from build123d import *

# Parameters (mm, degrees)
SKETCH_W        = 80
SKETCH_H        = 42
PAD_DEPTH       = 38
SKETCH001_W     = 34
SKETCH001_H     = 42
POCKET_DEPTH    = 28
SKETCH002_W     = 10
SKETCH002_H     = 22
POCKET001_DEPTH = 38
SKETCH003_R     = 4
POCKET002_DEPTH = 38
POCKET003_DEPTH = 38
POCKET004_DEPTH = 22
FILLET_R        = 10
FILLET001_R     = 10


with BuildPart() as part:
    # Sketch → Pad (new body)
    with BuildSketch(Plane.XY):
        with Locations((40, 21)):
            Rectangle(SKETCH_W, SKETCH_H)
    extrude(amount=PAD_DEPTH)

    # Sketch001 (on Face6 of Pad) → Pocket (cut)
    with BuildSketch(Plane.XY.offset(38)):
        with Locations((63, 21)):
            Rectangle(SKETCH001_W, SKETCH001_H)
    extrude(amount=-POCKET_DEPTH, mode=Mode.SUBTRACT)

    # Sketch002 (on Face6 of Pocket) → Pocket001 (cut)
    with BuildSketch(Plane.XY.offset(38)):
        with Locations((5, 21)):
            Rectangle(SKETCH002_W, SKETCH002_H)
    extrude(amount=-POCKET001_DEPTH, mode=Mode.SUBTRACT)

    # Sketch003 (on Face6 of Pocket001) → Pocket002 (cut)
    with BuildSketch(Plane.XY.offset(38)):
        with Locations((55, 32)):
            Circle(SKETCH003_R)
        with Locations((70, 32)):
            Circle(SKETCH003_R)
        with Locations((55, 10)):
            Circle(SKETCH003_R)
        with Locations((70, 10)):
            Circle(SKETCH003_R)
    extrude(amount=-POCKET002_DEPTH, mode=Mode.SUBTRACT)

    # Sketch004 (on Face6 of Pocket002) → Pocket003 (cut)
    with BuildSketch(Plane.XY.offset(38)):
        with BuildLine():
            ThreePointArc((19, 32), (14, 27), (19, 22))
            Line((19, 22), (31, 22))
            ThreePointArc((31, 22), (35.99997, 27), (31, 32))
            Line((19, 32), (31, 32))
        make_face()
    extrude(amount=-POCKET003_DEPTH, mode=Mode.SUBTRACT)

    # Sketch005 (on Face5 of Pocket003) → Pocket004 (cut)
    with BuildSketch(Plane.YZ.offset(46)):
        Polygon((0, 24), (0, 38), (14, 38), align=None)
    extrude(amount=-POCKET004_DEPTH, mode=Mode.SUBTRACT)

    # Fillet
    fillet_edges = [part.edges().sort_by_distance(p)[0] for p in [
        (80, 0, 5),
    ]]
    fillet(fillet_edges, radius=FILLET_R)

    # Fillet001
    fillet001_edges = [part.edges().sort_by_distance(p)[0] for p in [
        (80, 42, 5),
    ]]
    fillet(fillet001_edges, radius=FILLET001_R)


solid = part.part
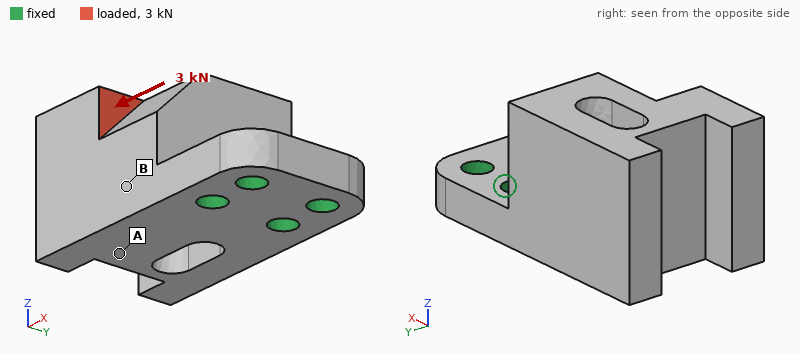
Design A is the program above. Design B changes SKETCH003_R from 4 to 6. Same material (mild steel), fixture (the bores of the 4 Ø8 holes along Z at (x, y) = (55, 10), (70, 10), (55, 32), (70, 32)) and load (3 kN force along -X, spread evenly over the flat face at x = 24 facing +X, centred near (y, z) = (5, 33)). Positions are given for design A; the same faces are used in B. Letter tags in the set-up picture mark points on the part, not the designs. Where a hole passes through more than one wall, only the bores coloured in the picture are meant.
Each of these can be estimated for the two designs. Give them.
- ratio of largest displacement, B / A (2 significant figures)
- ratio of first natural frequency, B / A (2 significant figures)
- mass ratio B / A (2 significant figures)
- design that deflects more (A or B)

0.80
1.1
0.96
A
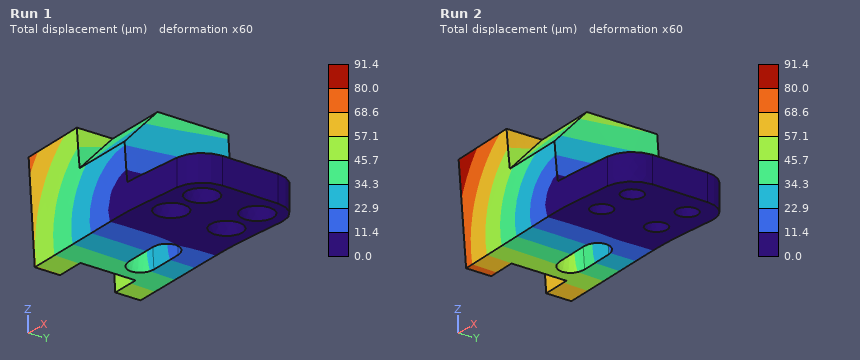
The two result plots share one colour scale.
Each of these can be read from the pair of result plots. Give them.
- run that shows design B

Run 1
